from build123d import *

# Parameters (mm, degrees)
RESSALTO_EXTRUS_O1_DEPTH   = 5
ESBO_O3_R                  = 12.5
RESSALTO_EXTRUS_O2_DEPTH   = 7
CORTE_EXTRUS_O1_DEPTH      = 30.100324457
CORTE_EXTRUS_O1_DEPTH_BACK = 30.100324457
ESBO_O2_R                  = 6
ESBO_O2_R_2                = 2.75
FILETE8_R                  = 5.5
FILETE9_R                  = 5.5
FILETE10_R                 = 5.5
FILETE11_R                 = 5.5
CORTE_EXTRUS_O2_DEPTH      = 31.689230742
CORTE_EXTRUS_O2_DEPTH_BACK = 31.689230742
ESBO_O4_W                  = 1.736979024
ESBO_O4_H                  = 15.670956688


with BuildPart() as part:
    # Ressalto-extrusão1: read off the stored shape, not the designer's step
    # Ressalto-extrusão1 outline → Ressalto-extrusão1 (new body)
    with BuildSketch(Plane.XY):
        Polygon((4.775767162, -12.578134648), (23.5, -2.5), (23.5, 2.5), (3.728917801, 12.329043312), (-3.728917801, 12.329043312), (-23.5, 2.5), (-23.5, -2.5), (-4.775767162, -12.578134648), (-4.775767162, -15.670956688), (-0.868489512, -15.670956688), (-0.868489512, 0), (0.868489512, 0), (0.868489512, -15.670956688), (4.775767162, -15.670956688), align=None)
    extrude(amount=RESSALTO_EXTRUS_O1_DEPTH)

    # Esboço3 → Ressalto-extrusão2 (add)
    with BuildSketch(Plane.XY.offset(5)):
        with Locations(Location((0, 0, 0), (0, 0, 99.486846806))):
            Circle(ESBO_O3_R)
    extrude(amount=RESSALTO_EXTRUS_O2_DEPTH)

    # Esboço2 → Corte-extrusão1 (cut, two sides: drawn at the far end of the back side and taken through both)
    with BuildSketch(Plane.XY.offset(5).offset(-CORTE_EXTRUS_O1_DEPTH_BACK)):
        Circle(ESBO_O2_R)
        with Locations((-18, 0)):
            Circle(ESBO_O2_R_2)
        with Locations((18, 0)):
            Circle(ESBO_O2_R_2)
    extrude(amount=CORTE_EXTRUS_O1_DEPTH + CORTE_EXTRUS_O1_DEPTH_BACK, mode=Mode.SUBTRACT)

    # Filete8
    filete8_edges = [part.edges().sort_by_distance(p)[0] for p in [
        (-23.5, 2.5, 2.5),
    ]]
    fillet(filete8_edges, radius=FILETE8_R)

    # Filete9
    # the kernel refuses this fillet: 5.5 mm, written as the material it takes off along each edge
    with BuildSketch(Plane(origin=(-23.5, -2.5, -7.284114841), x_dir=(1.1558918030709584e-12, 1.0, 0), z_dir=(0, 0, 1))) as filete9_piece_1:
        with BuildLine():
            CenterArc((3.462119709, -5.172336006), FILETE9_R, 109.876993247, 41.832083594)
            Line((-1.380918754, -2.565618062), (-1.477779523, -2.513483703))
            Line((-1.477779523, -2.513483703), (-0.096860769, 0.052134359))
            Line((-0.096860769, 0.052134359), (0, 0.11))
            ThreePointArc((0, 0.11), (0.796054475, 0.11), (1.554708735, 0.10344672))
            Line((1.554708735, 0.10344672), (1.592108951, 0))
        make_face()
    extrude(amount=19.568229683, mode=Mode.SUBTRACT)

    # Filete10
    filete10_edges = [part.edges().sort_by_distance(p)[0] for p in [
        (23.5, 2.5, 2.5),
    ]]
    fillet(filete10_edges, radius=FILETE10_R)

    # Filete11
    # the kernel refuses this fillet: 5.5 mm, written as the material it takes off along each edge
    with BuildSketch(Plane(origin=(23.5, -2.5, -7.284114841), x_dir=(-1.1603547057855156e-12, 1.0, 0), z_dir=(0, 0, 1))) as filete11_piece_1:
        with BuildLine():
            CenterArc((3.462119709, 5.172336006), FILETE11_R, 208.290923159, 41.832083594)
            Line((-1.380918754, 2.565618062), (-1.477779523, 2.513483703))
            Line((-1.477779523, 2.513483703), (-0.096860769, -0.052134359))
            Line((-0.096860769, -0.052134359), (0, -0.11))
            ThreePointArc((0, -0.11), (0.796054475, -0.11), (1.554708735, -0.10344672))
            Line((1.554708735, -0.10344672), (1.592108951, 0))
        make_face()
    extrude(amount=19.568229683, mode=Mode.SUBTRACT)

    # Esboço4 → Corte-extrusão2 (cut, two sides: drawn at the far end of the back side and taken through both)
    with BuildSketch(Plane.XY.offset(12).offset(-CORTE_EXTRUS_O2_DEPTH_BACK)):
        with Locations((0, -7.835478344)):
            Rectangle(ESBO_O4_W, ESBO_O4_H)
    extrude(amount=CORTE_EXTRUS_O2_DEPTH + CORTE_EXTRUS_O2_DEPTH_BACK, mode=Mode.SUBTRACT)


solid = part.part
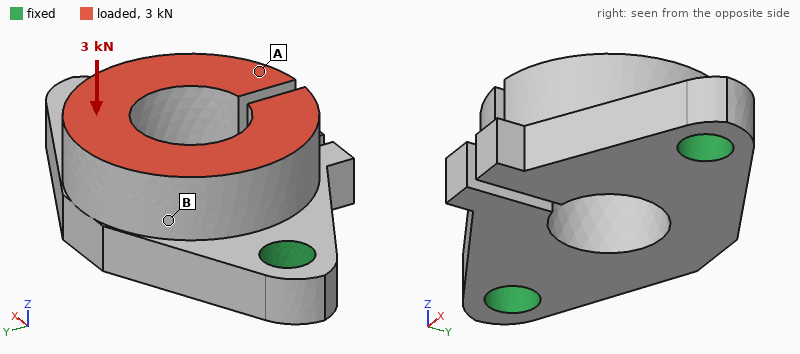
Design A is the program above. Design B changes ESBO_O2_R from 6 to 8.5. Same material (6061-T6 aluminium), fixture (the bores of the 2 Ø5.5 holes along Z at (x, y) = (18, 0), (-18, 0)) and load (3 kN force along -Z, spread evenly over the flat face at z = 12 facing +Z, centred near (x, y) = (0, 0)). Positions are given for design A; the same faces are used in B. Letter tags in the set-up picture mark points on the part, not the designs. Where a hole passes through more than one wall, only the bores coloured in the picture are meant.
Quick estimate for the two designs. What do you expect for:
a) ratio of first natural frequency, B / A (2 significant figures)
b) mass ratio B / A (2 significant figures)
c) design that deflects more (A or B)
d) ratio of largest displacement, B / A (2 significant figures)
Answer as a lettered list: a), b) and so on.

a) 0.99
b) 0.77
c) B
d) 1.6
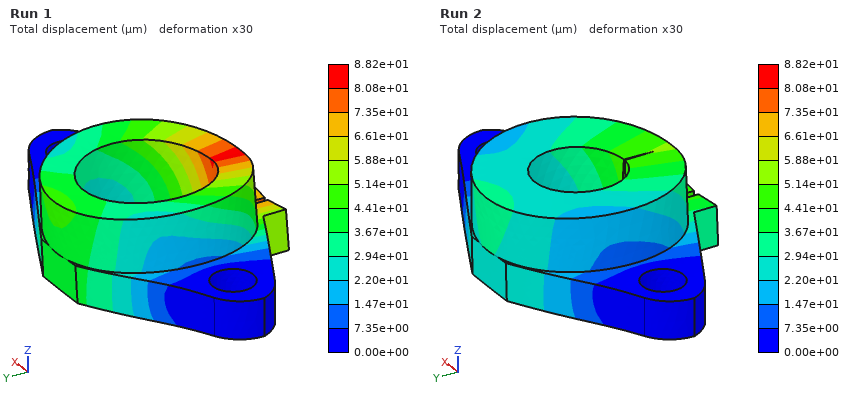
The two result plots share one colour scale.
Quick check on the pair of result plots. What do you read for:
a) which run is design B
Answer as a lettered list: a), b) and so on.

a) Run 1
